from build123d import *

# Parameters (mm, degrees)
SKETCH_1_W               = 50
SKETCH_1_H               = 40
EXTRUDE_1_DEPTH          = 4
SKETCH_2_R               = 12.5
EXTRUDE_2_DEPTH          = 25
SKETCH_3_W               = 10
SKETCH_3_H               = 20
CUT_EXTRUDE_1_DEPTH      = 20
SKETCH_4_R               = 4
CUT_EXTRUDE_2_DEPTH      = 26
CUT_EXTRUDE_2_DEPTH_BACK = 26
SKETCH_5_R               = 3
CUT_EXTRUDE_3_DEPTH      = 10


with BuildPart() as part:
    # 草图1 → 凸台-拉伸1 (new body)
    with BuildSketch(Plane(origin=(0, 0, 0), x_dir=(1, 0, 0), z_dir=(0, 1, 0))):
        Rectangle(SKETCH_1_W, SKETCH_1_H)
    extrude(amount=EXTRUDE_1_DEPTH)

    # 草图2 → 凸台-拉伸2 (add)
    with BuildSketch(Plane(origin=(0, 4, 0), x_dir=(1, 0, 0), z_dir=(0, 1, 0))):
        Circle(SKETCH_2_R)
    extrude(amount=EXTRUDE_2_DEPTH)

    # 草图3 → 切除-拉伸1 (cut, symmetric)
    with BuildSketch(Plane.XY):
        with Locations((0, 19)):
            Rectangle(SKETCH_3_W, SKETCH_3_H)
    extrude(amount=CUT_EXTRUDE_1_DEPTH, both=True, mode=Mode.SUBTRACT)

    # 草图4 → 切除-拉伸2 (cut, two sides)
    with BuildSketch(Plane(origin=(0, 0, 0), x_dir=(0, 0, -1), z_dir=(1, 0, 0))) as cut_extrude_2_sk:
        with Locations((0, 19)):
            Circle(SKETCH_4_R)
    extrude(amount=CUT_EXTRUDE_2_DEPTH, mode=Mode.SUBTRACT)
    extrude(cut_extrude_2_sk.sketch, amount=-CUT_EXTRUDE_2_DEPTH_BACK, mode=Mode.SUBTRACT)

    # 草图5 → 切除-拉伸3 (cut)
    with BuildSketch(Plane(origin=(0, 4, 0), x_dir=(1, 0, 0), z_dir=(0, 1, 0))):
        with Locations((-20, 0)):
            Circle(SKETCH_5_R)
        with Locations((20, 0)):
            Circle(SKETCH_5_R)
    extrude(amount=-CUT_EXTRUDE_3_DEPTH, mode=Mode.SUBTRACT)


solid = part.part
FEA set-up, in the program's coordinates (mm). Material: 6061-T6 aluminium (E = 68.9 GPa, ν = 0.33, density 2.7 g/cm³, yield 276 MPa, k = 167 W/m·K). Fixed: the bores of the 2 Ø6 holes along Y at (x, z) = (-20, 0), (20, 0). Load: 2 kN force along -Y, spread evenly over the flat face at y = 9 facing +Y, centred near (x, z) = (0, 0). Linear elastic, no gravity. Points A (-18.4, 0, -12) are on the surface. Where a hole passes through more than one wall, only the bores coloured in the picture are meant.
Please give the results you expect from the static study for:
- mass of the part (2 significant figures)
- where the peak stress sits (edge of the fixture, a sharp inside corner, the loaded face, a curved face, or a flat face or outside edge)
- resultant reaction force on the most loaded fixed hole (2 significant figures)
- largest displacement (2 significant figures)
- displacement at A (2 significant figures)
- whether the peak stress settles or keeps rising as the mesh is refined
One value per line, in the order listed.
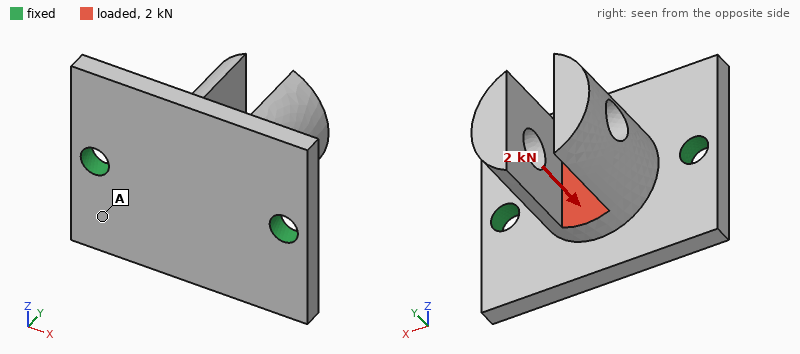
39 g
edge of the fixture
1.2 kN
27 µm
7.1 µm
keeps rising
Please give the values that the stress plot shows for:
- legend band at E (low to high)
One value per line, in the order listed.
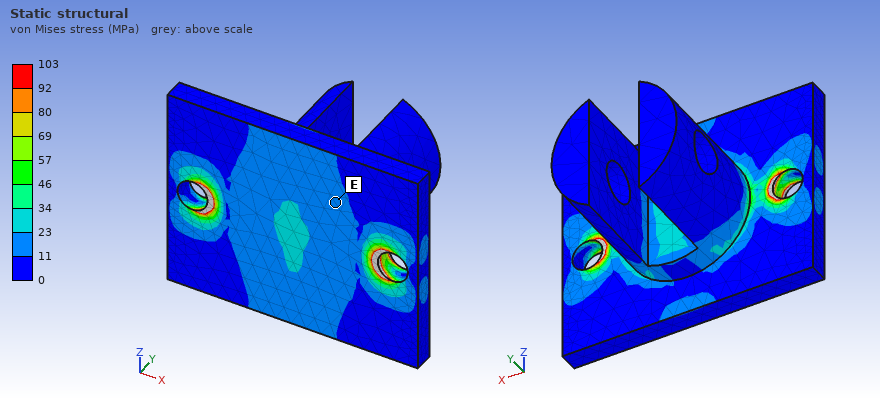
11 to 23 MPa
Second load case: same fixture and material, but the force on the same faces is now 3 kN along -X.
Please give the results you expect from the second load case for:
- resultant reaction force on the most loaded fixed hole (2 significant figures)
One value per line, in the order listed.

1.6 kN
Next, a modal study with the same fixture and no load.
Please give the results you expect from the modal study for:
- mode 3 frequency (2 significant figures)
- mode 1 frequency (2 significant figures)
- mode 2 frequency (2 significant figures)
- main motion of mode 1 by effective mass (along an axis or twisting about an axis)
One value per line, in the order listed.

8000 Hz
4000 Hz
7900 Hz
along Z
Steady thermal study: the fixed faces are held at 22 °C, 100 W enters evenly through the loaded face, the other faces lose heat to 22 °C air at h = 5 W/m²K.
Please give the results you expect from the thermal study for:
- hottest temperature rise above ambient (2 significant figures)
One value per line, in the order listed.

46 K
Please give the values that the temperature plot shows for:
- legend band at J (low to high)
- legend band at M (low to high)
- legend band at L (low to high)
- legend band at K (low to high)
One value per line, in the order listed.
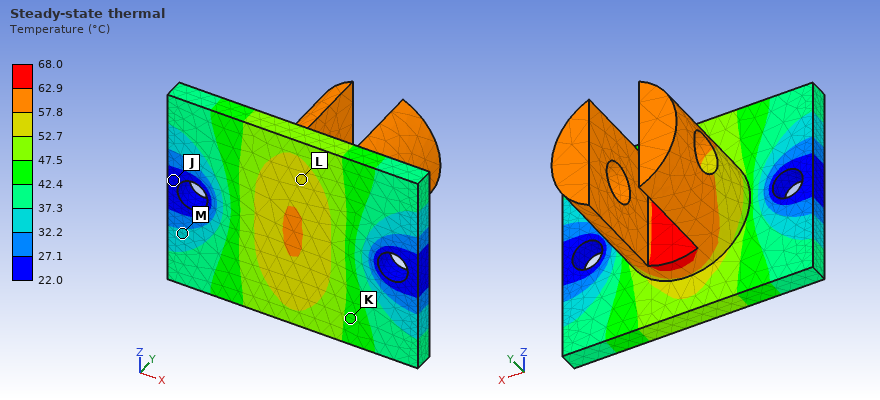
22.0 to 27.1 °C
32.2 to 37.3 °C
52.7 to 57.8 °C
42.4 to 47.5 °C
